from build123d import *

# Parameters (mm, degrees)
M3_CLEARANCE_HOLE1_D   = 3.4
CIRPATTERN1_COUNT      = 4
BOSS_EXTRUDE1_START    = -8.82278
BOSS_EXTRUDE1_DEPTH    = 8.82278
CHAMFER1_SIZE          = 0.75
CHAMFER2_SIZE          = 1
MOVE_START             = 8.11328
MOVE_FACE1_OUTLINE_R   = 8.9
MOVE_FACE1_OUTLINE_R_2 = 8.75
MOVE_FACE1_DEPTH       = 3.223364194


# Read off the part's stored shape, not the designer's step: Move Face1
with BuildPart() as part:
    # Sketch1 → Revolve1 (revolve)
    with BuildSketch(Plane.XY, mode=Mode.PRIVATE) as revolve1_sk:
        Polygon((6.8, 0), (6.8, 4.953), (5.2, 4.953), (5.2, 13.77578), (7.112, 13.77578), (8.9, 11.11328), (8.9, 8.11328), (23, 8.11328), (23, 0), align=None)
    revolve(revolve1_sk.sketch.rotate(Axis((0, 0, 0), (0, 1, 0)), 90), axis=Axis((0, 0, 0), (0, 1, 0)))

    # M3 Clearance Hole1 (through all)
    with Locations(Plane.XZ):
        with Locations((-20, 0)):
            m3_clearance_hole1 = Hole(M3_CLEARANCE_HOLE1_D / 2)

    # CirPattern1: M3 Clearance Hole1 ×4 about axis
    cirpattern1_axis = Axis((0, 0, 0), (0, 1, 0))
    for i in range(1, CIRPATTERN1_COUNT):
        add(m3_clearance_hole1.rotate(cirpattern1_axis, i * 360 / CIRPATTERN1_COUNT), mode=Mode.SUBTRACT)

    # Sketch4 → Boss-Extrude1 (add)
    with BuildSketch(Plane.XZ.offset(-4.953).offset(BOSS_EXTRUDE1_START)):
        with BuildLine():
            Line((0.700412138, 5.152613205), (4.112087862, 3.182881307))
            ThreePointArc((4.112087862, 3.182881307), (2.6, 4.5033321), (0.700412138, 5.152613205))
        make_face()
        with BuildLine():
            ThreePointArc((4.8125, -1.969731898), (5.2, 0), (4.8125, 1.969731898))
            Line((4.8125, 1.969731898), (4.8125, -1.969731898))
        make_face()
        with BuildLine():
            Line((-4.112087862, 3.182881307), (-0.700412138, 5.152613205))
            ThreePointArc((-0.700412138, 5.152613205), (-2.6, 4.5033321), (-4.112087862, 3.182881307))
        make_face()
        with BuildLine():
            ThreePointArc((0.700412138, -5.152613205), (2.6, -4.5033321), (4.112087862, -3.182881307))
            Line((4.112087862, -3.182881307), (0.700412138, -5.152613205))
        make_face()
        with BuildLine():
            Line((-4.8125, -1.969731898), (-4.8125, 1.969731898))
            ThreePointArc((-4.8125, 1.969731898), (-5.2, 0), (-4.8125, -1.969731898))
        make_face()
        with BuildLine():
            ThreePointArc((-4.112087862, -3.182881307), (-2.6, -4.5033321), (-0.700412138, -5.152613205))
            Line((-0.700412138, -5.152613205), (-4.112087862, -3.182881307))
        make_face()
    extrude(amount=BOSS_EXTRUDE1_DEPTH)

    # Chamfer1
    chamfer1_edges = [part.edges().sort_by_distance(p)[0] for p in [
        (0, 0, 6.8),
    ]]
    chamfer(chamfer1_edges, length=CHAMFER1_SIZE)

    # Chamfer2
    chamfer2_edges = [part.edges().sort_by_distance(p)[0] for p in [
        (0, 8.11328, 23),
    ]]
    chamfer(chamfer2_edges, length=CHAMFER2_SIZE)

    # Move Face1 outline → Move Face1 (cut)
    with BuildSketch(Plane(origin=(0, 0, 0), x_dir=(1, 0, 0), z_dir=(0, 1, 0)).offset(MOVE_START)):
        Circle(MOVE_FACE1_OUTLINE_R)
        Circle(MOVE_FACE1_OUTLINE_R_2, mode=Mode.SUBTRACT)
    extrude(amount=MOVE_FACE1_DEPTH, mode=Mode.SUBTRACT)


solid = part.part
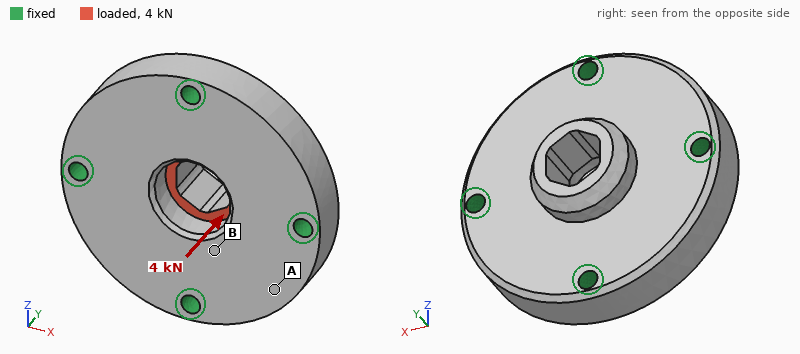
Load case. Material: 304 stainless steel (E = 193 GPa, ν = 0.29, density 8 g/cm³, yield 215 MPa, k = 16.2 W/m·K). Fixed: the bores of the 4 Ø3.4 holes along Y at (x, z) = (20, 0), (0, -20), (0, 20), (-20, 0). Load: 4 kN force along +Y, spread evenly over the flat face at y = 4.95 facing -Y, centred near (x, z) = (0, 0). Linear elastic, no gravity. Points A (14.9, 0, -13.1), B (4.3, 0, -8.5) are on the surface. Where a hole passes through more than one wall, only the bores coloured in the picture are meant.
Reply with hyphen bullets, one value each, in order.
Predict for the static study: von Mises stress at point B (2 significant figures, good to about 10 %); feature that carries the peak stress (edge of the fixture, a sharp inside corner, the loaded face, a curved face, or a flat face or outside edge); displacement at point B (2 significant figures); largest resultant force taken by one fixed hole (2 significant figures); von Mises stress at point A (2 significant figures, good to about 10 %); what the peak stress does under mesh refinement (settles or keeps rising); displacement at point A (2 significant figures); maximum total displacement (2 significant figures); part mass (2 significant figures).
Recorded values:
- 28 MPa
- edge of the fixture
- 3.8 µm
- 1.0 kN
- 14 MPa
- keeps rising
- 1.2 µm
- 6.1 µm
- 100 g
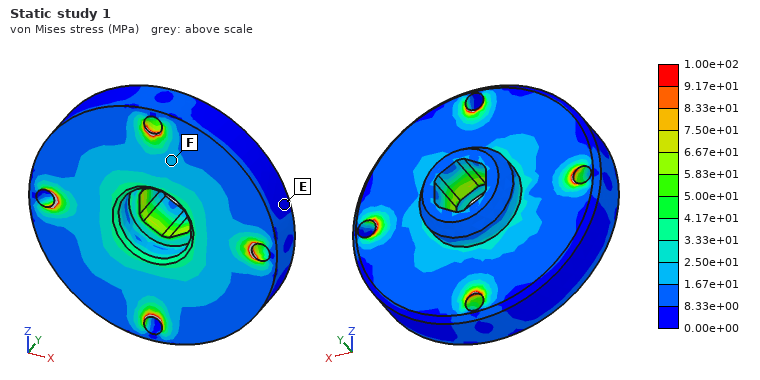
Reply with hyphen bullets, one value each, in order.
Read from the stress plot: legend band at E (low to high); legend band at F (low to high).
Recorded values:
- 0.00e+00 to 8.33e+00 MPa
- 1.67e+01 to 2.50e+01 MPa
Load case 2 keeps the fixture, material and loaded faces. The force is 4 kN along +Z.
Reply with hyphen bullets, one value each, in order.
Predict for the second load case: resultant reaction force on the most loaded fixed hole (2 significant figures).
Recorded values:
- 1.3 kN
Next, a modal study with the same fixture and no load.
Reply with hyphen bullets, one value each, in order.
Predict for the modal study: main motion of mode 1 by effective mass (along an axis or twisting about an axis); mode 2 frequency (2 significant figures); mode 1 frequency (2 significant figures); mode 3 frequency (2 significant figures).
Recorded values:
- along Y
- 32 kHz
- 27 kHz
- 32 kHz
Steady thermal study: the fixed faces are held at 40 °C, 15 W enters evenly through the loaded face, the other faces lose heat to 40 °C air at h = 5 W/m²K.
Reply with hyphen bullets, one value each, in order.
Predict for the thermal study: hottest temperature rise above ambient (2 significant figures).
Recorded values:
- 50 K
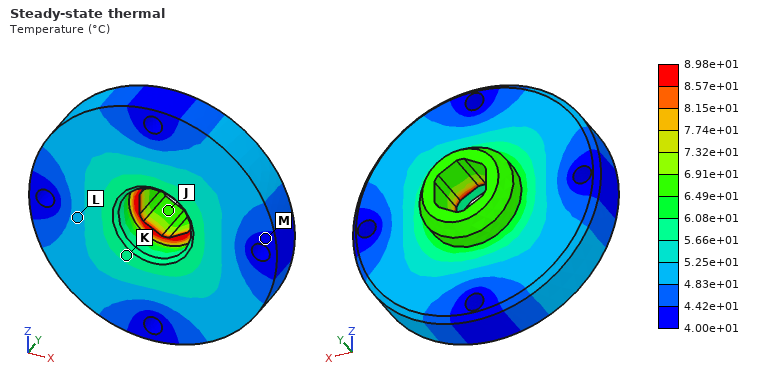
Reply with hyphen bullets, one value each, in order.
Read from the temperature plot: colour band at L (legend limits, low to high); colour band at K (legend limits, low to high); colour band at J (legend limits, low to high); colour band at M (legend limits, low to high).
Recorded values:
- 4.83e+01 to 5.25e+01 °C
- 5.66e+01 to 6.08e+01 °C
- 6.49e+01 to 6.91e+01 °C
- 4.00e+01 to 4.42e+01 °C
